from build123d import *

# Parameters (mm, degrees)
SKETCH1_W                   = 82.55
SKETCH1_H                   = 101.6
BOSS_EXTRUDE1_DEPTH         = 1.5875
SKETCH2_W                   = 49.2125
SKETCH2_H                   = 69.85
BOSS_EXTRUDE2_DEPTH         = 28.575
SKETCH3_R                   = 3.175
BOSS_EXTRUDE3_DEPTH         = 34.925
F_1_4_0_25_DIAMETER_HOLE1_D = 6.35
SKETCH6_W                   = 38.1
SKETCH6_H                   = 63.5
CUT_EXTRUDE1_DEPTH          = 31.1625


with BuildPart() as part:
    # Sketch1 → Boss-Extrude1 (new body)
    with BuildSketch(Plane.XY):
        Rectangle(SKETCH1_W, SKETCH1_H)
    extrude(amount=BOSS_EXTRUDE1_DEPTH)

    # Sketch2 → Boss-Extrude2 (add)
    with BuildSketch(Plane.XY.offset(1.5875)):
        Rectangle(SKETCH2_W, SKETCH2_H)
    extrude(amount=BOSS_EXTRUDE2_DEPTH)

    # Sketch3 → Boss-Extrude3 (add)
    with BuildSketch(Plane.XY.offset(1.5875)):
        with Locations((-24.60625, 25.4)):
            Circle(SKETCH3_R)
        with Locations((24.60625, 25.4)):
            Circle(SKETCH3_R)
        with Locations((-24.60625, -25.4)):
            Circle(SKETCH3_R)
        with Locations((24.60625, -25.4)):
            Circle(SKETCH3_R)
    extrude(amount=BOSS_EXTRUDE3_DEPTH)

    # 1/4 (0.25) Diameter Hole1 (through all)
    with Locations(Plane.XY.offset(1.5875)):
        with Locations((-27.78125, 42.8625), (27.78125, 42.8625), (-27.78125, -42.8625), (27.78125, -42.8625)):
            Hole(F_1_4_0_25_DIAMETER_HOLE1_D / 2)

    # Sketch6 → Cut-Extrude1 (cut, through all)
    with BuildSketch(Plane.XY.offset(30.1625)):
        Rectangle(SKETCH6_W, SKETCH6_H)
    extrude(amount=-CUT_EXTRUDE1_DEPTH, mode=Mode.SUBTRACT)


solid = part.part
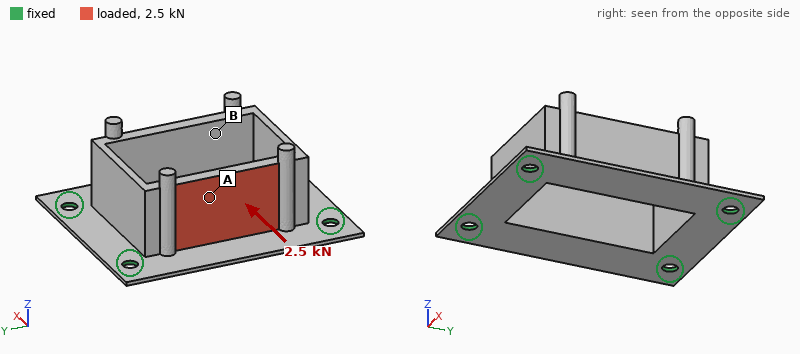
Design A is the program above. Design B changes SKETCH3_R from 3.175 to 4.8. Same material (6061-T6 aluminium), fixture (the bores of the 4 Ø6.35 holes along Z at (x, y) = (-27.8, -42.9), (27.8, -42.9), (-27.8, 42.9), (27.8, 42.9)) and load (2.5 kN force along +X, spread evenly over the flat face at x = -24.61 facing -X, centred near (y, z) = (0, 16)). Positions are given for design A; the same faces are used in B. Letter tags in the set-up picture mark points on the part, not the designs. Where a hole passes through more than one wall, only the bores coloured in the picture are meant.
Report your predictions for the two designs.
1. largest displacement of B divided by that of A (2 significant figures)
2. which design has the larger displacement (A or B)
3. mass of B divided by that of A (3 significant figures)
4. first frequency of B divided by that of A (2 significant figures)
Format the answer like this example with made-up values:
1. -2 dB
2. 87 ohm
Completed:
1. 0.90
2. A
3. 1.08
4. 0.96
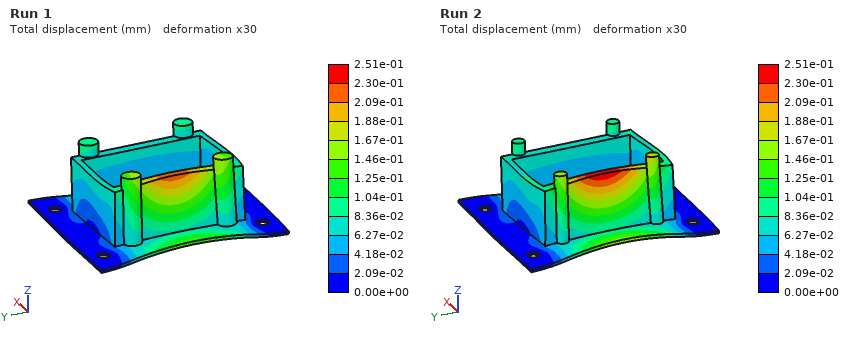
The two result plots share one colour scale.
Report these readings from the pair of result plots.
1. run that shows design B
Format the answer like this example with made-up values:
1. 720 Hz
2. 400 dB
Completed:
1. Run 1
